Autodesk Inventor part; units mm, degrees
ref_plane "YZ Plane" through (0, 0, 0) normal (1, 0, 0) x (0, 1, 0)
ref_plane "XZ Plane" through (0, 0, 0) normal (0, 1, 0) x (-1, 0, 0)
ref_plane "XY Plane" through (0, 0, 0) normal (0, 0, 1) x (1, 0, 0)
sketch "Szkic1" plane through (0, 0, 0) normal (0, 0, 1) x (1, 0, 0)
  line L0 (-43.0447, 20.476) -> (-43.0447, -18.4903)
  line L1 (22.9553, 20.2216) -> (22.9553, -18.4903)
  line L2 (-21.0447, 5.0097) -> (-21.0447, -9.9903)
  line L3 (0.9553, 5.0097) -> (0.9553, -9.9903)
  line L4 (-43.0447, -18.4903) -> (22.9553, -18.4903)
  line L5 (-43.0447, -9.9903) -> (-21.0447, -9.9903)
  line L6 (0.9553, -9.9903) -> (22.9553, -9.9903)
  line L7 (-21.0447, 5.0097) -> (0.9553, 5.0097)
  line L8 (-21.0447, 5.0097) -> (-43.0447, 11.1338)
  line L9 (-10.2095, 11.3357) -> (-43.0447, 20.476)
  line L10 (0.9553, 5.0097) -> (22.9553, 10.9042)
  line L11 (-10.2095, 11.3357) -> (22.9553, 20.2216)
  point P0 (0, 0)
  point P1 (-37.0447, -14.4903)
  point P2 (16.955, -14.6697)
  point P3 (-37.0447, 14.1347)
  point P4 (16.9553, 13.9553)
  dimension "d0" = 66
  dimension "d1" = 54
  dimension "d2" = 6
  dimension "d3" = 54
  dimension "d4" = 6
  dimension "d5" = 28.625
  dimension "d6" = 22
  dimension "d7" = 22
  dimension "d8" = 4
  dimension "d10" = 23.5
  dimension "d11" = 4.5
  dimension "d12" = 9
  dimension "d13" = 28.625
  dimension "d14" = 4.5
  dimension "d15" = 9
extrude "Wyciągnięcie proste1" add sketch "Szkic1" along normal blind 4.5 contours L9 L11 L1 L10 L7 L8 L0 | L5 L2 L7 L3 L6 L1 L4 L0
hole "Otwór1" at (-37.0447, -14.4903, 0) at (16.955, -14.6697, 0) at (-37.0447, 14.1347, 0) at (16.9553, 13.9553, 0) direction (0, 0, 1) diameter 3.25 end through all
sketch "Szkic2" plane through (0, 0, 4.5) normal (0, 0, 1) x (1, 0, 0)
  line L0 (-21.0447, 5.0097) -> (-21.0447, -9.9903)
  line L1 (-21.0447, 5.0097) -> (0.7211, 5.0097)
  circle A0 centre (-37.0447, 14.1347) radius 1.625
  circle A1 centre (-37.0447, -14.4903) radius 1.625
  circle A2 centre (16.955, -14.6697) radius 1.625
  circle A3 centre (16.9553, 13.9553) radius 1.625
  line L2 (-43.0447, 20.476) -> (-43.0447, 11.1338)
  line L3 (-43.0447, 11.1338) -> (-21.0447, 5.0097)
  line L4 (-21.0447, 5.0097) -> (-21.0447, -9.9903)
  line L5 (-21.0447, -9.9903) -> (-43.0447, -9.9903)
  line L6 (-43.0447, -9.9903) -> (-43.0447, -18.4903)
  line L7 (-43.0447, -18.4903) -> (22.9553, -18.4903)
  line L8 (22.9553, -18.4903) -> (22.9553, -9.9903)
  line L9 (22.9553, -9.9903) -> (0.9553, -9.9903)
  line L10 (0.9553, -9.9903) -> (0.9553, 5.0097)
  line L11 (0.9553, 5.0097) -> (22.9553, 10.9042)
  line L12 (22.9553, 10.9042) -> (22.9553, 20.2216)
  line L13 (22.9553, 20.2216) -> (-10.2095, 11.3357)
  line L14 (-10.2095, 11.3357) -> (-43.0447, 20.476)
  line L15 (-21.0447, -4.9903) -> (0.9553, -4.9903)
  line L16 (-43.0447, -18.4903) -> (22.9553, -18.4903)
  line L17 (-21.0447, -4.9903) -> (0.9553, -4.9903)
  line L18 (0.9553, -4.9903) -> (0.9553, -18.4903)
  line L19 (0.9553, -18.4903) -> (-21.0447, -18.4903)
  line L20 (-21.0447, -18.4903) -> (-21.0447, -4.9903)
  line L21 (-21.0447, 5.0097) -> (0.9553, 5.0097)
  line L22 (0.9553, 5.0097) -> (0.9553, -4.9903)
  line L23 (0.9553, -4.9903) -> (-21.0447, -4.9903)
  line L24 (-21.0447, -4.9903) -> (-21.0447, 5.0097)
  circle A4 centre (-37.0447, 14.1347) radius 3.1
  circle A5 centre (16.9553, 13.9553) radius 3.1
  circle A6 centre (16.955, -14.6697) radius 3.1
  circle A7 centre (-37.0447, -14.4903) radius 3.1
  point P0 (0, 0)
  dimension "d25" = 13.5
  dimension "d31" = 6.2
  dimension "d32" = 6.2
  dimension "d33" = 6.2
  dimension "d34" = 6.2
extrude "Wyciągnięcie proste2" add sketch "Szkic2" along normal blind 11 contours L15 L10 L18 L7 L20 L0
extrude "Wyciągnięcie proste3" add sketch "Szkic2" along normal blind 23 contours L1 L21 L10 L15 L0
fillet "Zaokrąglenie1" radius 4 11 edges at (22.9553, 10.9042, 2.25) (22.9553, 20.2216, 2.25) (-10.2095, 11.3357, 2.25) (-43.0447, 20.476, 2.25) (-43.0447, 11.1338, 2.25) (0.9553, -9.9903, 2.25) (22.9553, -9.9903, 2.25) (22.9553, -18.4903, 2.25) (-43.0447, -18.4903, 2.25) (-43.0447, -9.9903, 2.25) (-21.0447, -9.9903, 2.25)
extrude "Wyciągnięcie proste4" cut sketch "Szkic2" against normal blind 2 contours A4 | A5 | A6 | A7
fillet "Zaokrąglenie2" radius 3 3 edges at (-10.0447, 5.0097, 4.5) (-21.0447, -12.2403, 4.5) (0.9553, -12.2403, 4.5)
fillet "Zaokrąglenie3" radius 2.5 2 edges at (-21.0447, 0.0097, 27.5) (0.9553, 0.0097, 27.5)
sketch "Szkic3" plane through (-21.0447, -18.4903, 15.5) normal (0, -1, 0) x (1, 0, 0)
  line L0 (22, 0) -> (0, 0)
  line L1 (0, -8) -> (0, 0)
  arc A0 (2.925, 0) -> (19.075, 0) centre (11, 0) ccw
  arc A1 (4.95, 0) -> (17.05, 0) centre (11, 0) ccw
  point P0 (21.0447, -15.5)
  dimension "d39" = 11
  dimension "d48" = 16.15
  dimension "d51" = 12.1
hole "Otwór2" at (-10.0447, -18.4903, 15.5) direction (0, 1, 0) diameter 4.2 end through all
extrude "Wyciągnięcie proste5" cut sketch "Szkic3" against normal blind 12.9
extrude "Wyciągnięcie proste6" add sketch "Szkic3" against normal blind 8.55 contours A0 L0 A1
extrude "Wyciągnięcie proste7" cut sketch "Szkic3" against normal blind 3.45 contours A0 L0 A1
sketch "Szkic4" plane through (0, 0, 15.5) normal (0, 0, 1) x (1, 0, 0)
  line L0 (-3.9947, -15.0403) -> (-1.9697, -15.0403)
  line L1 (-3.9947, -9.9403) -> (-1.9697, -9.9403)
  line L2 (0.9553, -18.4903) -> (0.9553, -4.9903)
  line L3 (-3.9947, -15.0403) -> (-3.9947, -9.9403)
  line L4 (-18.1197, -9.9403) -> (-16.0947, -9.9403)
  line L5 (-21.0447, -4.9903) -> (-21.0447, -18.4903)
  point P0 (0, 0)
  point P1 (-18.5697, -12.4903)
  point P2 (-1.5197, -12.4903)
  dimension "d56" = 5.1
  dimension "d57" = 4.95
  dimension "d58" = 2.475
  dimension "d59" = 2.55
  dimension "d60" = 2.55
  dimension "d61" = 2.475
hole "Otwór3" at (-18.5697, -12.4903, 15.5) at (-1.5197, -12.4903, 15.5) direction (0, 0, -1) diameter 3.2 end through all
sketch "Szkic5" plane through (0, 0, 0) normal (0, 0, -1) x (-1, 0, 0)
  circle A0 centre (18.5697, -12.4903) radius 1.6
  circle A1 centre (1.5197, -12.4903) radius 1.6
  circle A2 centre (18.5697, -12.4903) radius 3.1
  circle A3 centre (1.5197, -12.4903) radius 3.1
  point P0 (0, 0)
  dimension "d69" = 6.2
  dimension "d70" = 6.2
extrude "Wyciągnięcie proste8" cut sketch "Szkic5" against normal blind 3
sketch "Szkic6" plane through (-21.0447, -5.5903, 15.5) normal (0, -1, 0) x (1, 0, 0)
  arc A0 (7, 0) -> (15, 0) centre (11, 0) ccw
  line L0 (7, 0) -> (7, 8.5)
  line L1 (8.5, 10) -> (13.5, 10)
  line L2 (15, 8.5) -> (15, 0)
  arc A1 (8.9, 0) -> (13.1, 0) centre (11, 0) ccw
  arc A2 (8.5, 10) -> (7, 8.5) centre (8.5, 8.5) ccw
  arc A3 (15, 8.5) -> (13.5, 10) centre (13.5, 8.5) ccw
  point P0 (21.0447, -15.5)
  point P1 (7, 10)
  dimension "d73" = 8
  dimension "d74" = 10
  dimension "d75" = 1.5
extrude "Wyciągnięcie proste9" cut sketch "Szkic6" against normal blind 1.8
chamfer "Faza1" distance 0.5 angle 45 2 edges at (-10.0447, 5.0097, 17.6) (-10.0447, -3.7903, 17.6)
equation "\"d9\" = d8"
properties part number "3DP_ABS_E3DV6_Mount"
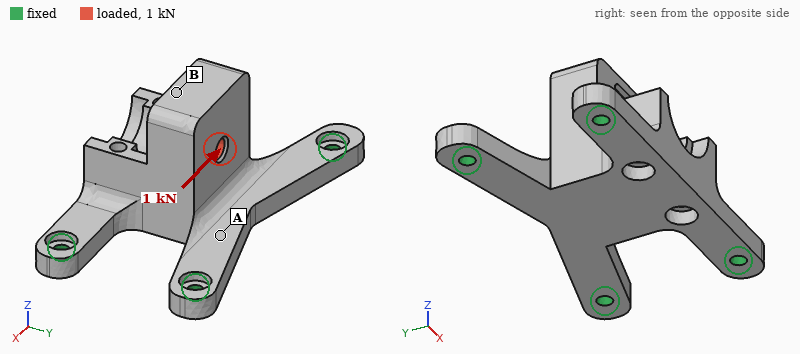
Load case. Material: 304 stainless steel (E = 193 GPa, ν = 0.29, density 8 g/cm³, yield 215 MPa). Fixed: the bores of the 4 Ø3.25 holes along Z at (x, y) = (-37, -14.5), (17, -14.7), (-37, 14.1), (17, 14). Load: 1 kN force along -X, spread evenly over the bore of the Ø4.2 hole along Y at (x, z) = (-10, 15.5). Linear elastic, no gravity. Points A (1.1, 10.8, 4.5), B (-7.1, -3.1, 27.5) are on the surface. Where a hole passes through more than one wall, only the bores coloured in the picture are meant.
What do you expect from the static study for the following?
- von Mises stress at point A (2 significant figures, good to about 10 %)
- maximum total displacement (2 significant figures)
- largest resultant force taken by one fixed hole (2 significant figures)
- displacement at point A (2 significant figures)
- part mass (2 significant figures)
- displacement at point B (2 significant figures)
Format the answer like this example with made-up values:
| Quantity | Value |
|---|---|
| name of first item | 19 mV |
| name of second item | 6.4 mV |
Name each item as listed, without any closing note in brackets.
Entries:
| Quantity | Value |
|---|---|
| von Mises stress at point A | 34 MPa |
| maximum total displacement | 17 µm |
| largest resultant force taken by one fixed hole | 340 N |
| displacement at point A | 4.0 µm |
| part mass | 100 g |
| displacement at point B | 16 µm |
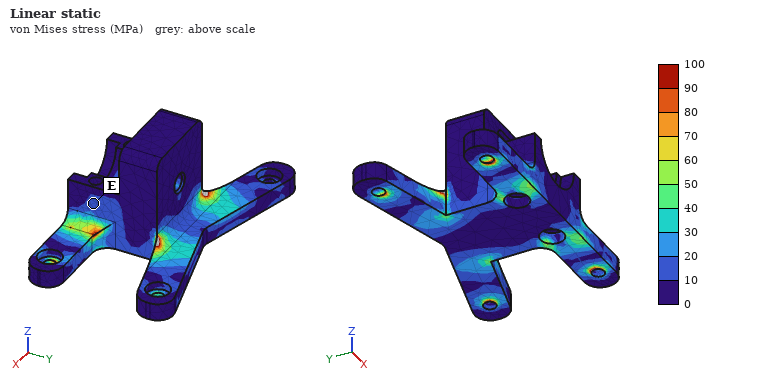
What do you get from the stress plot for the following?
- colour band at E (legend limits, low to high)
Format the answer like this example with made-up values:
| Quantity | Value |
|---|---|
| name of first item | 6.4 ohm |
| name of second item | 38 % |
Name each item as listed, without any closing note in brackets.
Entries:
| Quantity | Value |
|---|---|
| colour band at E | 10 to 20 MPa |
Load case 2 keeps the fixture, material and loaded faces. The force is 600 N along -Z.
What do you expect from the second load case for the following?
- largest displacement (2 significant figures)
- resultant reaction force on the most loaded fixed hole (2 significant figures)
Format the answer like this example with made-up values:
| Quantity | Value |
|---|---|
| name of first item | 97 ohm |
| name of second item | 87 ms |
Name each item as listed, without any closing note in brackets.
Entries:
| Quantity | Value |
|---|---|
| largest displacement | 15 µm |
| resultant reaction force on the most loaded fixed hole | 270 N |
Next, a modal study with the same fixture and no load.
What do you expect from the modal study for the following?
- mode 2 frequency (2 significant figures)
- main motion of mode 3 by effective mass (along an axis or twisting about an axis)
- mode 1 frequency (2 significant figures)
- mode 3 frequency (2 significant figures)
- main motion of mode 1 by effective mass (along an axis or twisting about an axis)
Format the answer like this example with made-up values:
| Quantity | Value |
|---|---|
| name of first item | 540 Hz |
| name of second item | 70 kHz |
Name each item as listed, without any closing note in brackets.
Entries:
| Quantity | Value |
|---|---|
| mode 2 frequency | 4500 Hz |
| main motion of mode 3 by effective mass | along X |
| mode 1 frequency | 4100 Hz |
| mode 3 frequency | 6400 Hz |
| main motion of mode 1 by effective mass | along Z |
